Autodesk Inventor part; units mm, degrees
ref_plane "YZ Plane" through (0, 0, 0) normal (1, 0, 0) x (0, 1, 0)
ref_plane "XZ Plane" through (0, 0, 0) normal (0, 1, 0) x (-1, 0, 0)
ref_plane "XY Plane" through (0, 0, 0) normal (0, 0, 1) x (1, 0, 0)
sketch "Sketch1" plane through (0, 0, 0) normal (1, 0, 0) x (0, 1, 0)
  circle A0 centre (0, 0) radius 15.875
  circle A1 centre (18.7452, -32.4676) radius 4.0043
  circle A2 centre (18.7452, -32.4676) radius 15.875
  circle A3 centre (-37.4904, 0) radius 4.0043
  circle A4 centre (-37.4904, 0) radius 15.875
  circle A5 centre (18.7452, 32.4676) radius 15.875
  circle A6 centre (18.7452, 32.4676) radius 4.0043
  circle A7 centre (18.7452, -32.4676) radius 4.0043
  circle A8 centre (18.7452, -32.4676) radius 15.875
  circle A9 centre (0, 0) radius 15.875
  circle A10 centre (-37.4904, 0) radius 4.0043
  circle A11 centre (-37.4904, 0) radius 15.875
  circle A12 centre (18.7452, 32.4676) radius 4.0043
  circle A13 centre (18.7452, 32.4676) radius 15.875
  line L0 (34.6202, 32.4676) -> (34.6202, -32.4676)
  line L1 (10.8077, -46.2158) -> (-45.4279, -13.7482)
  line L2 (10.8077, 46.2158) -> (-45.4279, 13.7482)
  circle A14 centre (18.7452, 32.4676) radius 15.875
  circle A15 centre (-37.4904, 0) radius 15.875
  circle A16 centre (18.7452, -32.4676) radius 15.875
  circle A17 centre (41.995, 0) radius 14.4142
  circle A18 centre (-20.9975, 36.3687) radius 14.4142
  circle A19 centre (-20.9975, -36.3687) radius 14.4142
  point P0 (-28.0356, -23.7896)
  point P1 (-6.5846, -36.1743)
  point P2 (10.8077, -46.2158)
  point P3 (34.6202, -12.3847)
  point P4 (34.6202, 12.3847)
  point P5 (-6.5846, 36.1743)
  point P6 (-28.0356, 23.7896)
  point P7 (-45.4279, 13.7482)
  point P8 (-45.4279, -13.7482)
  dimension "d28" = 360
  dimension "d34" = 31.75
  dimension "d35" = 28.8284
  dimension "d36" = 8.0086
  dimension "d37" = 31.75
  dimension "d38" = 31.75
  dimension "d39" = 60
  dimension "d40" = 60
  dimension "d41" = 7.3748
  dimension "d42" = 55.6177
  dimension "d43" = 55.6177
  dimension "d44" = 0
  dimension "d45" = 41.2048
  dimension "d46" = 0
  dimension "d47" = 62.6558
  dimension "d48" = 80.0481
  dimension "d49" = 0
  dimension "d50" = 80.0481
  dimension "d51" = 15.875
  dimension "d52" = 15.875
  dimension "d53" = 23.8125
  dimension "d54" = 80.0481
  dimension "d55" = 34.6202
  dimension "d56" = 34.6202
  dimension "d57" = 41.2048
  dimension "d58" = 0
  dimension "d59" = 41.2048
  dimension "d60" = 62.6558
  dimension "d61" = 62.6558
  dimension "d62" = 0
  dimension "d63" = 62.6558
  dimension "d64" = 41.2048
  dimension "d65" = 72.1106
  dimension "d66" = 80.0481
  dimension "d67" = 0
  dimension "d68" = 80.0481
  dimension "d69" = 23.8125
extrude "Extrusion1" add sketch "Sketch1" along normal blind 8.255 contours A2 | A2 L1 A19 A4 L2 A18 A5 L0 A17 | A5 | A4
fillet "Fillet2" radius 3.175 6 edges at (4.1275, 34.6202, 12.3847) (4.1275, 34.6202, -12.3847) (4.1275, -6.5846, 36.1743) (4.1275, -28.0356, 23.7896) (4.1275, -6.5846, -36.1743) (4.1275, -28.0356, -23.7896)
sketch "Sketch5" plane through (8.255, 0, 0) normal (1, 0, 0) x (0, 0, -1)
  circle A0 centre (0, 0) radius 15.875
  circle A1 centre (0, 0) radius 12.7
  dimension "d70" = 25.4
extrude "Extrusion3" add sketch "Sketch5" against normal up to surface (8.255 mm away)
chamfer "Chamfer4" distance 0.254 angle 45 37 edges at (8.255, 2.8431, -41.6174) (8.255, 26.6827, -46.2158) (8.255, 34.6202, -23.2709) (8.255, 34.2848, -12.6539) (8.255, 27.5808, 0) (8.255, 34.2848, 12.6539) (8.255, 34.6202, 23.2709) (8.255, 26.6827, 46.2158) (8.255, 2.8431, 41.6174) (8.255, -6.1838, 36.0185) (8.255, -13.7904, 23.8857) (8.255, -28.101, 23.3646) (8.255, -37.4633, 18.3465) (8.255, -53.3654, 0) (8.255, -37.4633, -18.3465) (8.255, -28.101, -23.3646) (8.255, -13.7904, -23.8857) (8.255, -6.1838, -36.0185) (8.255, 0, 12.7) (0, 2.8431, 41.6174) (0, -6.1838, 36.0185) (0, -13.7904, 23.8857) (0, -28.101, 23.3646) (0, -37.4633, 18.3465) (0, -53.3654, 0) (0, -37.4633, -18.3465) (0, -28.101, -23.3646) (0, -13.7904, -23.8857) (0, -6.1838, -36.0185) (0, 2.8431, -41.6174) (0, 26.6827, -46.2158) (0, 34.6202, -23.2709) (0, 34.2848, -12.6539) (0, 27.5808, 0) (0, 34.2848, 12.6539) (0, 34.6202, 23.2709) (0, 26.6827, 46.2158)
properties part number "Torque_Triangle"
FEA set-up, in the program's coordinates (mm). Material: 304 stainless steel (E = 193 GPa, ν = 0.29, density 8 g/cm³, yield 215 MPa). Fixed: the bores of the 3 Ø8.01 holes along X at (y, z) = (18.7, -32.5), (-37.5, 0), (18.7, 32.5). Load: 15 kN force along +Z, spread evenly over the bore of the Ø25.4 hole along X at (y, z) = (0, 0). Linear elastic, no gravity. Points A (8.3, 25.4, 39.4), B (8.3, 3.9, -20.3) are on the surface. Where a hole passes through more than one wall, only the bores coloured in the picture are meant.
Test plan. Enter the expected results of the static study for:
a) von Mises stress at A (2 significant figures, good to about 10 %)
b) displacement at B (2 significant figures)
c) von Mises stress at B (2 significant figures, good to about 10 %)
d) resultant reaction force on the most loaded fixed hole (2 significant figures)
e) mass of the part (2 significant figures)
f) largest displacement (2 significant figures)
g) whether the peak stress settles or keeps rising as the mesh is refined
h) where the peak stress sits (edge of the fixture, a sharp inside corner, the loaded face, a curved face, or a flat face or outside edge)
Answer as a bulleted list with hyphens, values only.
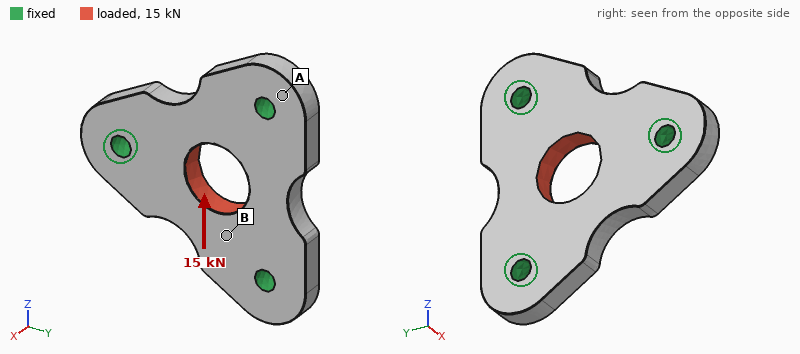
- 13 MPa
- 5.2 µm
- 33 MPa
- 5.8 kN
- 310 g
- 10 µm
- keeps rising
- edge of the fixture
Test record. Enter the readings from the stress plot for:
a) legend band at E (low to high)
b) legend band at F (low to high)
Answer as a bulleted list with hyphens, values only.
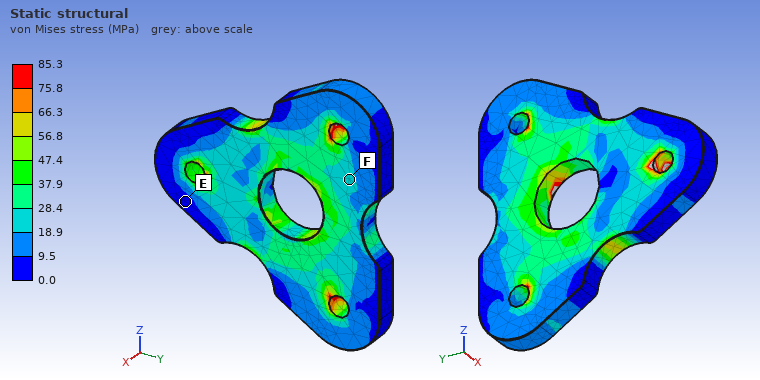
- 0.0 to 9.5 MPa
- 18.9 to 28.4 MPa
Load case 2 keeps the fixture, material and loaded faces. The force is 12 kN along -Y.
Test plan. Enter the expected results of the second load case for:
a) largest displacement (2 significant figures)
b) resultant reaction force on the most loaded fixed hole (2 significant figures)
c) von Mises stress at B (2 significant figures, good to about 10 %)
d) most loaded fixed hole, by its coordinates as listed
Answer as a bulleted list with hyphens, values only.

- 8.9 µm
- 5.1 kN
- 14 MPa
- (-37.5, 0)
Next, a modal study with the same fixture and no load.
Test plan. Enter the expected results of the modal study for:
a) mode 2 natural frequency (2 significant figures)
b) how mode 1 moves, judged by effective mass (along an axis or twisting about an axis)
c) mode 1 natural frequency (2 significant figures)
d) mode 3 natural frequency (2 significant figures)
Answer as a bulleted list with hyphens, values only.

- 11 kHz
- along X
- 9700 Hz
- 11 kHz
